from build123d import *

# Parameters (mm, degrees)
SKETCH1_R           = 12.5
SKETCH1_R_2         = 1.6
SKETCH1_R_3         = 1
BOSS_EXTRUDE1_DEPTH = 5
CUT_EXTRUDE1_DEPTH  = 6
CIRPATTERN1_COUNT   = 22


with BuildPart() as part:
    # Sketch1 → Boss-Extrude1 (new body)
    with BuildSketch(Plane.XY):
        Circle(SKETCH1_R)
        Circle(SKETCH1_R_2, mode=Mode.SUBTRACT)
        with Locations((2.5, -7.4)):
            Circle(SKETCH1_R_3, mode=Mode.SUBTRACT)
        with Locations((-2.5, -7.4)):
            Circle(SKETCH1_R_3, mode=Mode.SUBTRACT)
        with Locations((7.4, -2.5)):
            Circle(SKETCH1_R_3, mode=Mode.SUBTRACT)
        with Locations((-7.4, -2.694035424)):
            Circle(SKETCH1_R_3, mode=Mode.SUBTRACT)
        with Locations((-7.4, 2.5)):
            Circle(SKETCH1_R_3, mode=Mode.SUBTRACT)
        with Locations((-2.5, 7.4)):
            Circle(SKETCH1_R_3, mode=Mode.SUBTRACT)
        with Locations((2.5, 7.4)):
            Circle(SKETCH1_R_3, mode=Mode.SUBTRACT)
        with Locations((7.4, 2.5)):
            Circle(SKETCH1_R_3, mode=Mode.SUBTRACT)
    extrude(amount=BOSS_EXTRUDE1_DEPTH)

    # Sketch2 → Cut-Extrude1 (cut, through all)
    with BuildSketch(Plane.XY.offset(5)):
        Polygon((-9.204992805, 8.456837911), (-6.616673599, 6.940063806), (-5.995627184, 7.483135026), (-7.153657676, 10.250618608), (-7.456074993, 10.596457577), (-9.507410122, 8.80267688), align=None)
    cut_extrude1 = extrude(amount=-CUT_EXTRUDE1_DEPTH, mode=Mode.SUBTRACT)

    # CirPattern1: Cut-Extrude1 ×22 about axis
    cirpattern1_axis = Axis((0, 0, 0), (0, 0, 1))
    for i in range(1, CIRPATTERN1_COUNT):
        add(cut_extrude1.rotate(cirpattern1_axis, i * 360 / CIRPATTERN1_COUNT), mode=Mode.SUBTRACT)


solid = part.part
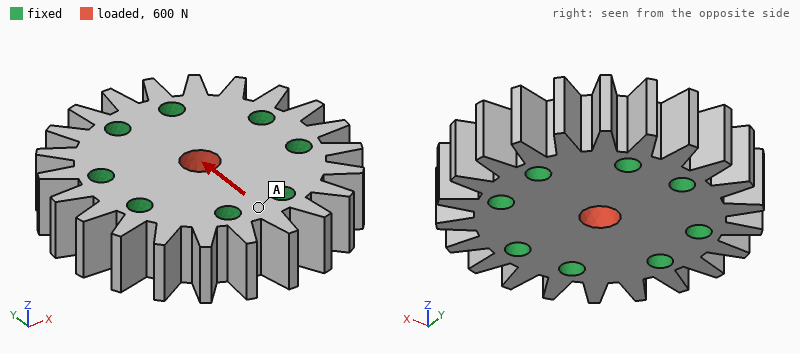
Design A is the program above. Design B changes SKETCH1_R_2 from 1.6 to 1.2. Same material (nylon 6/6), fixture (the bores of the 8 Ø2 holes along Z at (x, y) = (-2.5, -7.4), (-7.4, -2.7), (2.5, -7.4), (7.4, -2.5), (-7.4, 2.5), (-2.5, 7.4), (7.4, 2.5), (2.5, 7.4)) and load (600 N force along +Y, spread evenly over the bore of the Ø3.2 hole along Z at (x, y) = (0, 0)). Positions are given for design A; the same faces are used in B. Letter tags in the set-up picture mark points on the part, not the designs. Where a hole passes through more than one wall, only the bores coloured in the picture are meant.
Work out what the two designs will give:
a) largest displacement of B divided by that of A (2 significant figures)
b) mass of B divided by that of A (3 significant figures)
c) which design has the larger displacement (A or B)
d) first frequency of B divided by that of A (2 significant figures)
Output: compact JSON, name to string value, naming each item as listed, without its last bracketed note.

{"largest displacement of B divided by that of A": "1.2", "mass of B divided by that of A": "1.01", "which design has the larger displacement": "B", "first frequency of B divided by that of A": "0.99"}
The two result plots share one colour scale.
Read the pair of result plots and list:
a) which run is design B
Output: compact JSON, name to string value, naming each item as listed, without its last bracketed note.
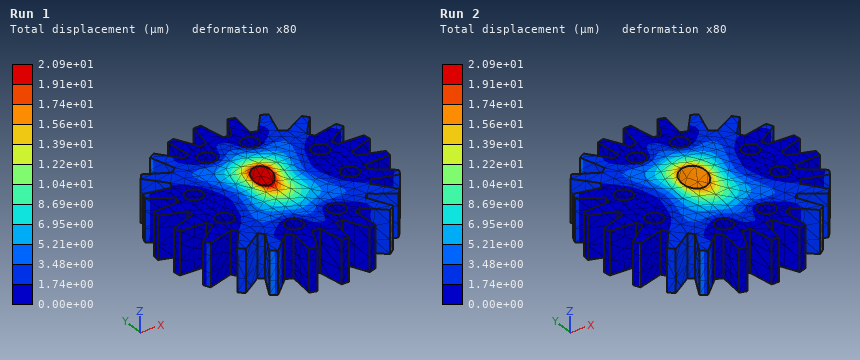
{"which run is design B": "Run 1"}
